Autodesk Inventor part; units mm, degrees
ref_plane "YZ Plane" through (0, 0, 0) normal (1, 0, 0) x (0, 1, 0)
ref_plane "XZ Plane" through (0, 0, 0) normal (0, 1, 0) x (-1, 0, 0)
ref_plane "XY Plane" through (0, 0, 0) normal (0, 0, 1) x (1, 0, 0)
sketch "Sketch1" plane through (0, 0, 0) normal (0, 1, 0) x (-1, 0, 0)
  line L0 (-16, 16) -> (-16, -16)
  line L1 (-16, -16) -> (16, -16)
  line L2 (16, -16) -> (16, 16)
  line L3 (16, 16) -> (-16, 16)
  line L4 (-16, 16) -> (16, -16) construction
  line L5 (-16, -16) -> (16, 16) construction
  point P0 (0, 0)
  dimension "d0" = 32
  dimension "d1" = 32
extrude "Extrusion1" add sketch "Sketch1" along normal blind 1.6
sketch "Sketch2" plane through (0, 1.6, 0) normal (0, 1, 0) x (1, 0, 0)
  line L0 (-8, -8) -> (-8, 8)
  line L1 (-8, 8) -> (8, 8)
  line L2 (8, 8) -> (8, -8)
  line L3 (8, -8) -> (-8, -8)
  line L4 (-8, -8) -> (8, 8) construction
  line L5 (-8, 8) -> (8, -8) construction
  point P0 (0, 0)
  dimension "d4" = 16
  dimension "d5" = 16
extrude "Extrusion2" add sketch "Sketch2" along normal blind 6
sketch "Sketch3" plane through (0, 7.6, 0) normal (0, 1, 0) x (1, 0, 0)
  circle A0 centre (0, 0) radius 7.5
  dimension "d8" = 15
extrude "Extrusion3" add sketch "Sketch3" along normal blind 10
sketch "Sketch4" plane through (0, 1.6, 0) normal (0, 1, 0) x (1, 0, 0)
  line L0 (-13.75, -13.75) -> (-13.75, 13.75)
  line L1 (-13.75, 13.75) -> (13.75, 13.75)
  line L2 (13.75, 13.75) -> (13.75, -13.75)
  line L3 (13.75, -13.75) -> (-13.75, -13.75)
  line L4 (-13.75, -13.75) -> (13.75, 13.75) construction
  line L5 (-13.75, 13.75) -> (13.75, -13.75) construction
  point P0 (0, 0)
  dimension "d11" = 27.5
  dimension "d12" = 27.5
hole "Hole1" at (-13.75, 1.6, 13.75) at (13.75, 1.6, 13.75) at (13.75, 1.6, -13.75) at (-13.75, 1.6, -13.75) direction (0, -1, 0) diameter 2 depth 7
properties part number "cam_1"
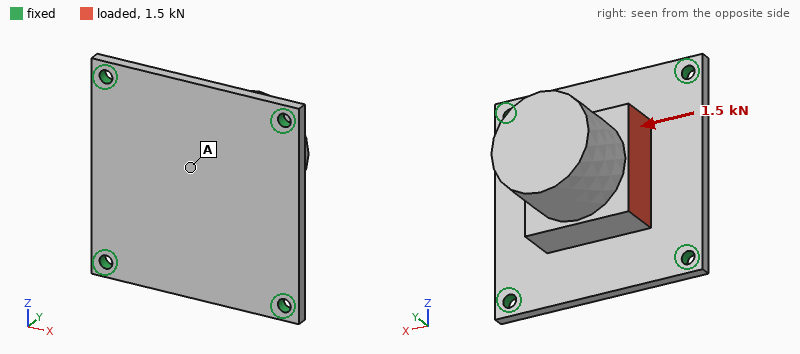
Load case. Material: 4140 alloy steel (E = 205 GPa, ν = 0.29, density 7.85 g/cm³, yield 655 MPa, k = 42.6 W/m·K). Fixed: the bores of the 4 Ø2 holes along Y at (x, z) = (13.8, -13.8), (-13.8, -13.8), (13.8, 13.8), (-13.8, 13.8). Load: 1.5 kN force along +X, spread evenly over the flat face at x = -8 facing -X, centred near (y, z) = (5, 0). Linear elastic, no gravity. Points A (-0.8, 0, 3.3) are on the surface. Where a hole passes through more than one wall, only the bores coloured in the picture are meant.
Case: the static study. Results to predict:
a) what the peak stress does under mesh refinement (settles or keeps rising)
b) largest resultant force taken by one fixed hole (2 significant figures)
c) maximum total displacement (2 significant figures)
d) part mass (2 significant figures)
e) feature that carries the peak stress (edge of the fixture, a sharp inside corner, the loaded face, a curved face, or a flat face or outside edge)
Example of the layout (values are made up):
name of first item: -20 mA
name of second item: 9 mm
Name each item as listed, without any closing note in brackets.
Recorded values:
what the peak stress does under mesh refinement: keeps rising
largest resultant force taken by one fixed hole: 440 N
maximum total displacement: 26 µm
part mass: 39 g
feature that carries the peak stress: edge of the fixture
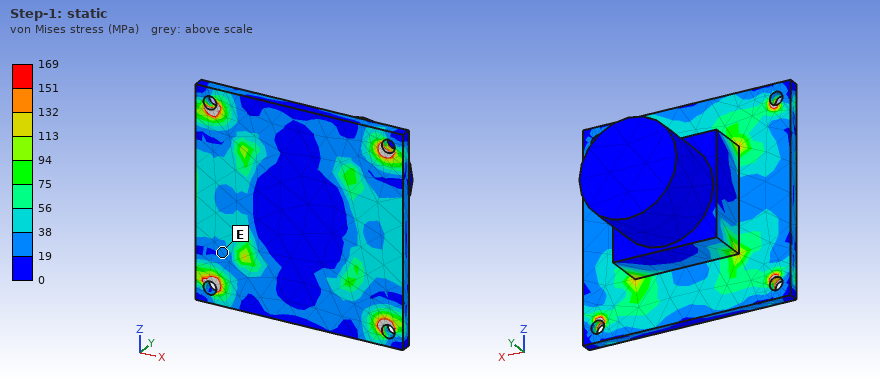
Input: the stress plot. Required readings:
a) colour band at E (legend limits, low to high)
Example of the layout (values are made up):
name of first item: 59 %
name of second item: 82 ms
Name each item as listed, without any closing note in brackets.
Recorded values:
colour band at E: 19 to 38 MPa
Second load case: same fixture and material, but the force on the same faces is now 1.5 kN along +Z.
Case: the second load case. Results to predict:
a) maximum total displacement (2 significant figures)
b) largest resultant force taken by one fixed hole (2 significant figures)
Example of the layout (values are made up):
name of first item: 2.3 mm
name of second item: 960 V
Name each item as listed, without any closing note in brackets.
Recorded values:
maximum total displacement: 26 µm
largest resultant force taken by one fixed hole: 520 N
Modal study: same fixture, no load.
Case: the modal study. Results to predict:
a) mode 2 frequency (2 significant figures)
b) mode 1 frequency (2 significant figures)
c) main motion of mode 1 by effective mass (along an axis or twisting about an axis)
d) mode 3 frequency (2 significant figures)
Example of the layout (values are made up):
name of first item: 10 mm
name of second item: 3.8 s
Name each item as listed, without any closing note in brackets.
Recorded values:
mode 2 frequency: 5800 Hz
mode 1 frequency: 5000 Hz
main motion of mode 1 by effective mass: along Y
mode 3 frequency: 5800 Hz
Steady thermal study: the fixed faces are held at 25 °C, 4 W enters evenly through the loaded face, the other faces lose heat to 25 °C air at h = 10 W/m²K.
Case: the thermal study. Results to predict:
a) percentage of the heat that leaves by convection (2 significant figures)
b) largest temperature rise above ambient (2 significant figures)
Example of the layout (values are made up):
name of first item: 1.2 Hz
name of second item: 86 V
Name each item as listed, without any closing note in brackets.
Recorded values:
percentage of the heat that leaves by convection: 8.1 %
largest temperature rise above ambient: 19 K
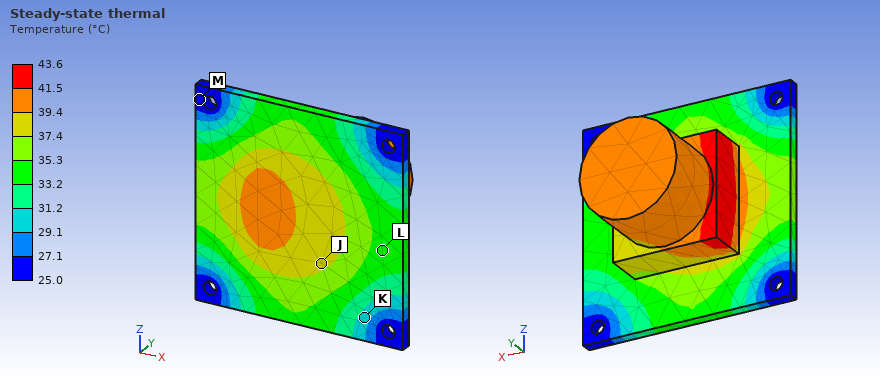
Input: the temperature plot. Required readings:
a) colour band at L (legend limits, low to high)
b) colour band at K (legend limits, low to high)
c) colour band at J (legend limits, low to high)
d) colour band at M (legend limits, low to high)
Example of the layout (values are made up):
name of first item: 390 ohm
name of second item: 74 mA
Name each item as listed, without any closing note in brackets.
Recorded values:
colour band at L: 33.2 to 35.3 °C
colour band at K: 29.1 to 31.2 °C
colour band at J: 37.4 to 39.4 °C
colour band at M: 25.0 to 27.1 °C
